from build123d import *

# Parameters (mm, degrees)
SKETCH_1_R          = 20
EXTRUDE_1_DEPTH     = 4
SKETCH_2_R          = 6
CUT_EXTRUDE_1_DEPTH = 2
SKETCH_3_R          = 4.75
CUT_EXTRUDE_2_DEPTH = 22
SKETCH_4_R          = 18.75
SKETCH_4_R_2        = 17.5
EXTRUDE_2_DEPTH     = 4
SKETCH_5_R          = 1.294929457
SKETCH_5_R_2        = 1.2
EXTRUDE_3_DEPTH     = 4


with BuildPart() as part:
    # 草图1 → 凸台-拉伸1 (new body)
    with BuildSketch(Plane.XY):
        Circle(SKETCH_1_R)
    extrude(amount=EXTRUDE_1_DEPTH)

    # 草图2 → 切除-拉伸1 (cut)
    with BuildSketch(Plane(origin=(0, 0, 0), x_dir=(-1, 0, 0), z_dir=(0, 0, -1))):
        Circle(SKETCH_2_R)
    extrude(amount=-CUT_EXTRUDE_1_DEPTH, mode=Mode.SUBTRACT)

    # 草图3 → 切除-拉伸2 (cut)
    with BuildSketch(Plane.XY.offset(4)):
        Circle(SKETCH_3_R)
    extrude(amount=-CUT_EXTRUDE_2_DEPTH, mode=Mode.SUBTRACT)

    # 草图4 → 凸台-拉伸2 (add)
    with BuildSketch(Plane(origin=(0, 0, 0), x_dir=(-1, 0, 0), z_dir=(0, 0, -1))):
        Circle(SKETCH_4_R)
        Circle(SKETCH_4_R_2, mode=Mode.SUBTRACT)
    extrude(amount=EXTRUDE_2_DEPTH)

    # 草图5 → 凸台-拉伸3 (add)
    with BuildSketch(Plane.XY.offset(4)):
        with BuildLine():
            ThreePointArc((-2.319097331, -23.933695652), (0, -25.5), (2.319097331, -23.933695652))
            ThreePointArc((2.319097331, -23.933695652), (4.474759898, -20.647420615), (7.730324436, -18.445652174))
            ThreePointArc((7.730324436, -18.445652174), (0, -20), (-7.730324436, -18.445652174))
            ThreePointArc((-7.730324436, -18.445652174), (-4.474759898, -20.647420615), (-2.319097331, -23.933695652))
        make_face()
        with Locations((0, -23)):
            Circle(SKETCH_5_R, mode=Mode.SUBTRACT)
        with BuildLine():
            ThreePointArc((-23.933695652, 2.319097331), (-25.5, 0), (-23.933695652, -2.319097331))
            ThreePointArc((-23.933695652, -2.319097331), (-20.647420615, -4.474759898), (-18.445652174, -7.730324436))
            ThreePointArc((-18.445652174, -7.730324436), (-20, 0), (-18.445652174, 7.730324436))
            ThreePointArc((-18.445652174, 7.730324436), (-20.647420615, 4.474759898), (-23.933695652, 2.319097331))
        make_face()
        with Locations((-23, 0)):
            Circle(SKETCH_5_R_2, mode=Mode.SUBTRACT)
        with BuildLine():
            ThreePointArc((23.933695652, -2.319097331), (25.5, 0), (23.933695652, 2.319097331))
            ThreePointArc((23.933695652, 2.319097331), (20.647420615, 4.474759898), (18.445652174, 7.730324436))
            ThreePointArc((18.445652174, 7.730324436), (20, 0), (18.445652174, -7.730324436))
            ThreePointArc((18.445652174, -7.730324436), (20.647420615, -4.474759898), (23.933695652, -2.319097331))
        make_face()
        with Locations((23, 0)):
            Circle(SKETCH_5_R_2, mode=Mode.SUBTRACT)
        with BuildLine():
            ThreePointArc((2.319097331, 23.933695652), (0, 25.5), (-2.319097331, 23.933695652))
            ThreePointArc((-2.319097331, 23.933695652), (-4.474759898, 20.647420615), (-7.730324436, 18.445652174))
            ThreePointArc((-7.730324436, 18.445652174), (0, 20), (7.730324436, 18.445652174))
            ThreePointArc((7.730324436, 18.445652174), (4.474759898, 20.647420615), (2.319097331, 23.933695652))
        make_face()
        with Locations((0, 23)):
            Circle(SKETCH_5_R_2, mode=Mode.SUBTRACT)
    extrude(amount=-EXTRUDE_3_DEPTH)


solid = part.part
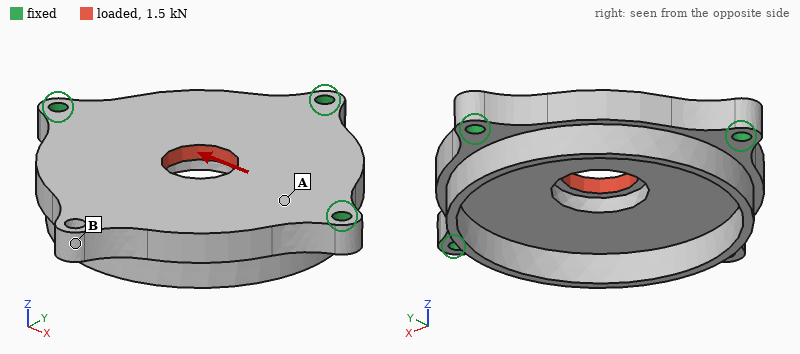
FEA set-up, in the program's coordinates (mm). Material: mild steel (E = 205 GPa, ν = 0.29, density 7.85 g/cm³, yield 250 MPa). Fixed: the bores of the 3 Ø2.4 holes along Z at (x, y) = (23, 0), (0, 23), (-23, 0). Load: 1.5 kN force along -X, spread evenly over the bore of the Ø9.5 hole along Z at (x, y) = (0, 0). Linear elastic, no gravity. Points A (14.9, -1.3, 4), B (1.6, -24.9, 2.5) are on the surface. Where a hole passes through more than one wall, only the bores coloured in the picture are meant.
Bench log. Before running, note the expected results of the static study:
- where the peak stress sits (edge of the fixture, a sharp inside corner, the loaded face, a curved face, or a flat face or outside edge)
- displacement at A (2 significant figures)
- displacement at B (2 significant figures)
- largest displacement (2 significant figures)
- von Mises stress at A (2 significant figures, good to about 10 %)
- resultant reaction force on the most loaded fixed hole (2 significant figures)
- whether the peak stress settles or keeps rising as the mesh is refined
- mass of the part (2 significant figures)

edge of the fixture
0.80 µm
1.1 µm
1.9 µm
20 MPa
670 N
keeps rising
45 g
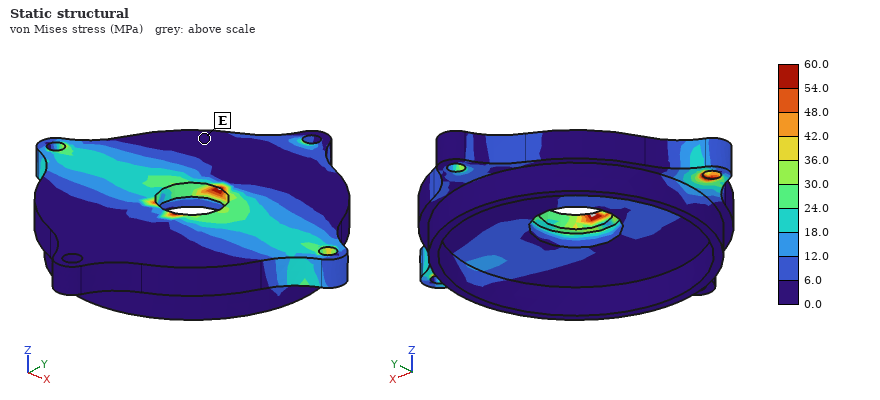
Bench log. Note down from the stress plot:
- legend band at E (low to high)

0.0 to 6.0 MPa
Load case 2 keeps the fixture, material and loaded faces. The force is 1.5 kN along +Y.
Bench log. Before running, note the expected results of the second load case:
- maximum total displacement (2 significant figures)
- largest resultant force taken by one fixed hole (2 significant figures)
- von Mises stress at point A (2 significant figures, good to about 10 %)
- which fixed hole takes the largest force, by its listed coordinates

7.5 µm
780 N
7.7 MPa
(0, 23)
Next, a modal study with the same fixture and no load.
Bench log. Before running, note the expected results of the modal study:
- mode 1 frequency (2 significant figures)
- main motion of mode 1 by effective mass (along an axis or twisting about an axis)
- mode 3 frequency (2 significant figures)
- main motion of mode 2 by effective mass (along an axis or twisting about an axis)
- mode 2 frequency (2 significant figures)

4900 Hz
along Z
16 kHz
along Z
14 kHz
